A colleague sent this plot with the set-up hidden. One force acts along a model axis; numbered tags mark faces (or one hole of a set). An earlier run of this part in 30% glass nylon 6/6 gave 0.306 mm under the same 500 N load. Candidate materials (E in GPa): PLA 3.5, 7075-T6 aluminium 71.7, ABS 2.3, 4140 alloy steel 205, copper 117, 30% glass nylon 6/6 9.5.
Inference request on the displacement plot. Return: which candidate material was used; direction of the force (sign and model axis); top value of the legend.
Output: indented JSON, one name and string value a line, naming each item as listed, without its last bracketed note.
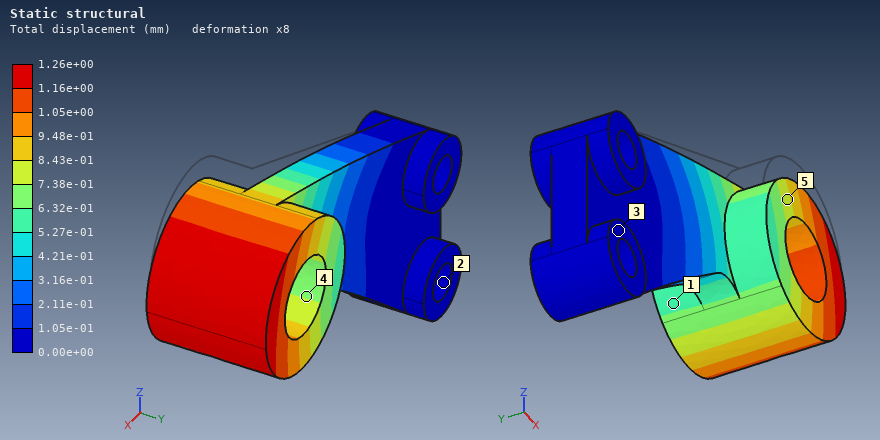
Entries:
{
  "which candidate material was used": "ABS",
  "direction of the force": "-Z",
  "top value of the legend": "1.26e+00 mm"
}
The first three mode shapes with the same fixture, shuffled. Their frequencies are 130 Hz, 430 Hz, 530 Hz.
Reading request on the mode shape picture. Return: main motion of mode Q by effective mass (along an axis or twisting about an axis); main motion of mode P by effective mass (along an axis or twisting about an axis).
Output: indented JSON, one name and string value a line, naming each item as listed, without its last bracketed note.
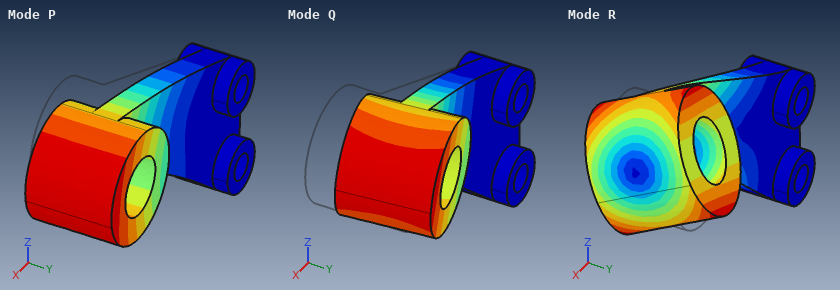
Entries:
{
  "main motion of mode Q by effective mass": "along Y",
  "main motion of mode P by effective mass": "along Z"
}
